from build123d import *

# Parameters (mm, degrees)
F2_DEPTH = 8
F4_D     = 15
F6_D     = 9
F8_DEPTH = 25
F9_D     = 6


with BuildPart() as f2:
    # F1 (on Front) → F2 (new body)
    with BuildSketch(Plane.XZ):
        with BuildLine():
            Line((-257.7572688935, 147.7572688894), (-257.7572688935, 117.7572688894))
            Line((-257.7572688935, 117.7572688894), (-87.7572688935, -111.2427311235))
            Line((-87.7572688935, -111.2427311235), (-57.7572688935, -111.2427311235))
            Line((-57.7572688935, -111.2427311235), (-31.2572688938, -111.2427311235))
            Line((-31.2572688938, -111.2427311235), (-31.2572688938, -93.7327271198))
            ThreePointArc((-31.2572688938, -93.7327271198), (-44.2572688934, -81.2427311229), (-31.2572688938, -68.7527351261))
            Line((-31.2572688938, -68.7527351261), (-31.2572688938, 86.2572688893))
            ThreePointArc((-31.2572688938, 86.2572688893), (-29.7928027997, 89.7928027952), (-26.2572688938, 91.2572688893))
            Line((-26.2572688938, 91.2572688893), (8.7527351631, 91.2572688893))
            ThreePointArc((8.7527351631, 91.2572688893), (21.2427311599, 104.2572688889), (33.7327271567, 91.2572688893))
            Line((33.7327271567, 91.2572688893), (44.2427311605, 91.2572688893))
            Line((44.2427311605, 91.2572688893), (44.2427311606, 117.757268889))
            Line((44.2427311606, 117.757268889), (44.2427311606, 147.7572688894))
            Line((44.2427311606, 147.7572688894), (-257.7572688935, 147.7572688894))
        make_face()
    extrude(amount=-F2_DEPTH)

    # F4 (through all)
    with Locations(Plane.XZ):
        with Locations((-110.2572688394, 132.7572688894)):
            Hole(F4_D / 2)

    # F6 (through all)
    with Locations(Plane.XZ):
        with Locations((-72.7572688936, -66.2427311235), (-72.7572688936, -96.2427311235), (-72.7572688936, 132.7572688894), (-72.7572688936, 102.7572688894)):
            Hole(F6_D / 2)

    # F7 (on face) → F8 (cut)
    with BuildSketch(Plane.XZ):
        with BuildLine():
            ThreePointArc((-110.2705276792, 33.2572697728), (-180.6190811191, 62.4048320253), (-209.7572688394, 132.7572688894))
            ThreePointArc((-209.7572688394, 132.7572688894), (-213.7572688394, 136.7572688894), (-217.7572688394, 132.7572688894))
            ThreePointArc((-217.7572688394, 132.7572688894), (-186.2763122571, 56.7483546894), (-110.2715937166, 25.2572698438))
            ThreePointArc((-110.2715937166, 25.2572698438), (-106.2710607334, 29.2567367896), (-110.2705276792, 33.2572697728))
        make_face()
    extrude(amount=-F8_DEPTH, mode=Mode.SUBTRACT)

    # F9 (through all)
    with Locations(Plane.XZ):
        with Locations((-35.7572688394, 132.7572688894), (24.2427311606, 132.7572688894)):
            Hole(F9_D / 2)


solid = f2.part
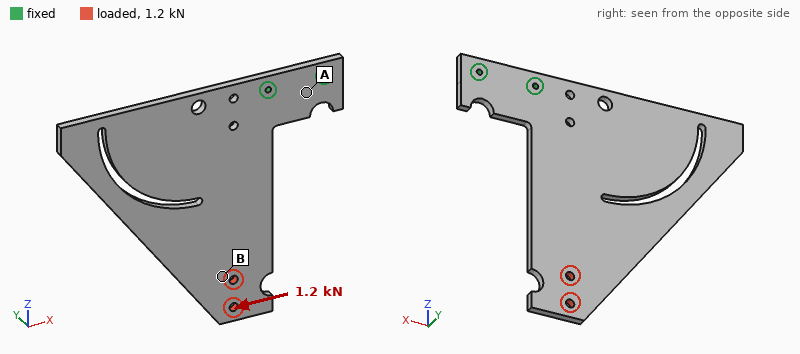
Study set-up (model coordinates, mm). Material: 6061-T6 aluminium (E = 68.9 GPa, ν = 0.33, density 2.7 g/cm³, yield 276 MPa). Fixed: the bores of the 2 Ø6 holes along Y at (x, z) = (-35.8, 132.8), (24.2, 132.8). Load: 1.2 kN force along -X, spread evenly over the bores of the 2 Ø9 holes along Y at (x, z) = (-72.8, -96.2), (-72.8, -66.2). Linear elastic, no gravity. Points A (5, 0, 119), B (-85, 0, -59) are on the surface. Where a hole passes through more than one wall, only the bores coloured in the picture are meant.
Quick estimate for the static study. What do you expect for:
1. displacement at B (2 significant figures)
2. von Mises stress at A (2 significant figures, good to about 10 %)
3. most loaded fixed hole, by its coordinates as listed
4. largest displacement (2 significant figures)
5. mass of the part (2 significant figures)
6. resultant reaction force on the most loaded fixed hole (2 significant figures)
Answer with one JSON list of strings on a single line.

["0.34 mm", "24 MPa", "(24.2, 132.8)", "0.44 mm", "890 g", "4.9 kN"]
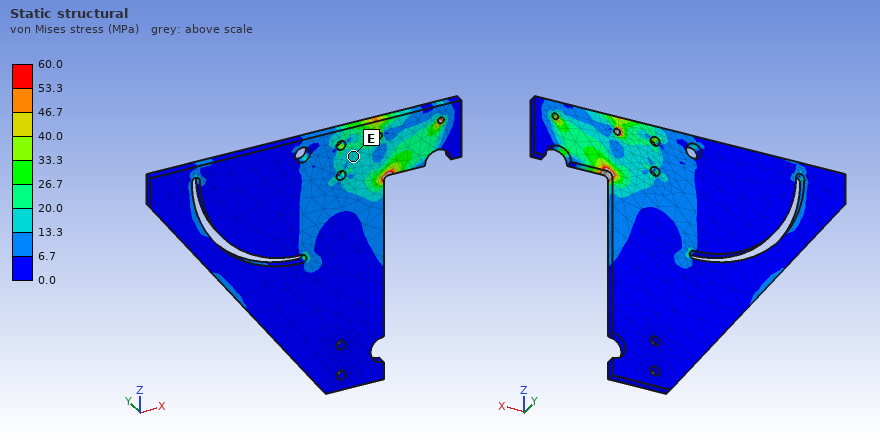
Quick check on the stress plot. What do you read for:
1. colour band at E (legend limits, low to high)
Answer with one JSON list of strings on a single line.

["13.3 to 20.0 MPa"]
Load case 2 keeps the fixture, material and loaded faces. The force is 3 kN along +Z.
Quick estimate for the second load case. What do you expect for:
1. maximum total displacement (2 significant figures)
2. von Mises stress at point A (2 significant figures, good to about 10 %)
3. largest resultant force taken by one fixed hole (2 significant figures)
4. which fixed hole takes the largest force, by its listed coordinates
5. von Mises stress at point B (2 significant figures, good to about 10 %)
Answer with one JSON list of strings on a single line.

["0.17 mm", "9.7 MPa", "4.8 kN", "(-35.8, 132.8)", "6.2 MPa"]
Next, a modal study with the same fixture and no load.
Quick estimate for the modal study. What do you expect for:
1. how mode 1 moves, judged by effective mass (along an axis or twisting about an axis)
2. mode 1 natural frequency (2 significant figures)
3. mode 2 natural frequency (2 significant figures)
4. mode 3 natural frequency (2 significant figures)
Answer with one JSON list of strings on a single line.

["along Y", "91 Hz", "140 Hz", "470 Hz"]
